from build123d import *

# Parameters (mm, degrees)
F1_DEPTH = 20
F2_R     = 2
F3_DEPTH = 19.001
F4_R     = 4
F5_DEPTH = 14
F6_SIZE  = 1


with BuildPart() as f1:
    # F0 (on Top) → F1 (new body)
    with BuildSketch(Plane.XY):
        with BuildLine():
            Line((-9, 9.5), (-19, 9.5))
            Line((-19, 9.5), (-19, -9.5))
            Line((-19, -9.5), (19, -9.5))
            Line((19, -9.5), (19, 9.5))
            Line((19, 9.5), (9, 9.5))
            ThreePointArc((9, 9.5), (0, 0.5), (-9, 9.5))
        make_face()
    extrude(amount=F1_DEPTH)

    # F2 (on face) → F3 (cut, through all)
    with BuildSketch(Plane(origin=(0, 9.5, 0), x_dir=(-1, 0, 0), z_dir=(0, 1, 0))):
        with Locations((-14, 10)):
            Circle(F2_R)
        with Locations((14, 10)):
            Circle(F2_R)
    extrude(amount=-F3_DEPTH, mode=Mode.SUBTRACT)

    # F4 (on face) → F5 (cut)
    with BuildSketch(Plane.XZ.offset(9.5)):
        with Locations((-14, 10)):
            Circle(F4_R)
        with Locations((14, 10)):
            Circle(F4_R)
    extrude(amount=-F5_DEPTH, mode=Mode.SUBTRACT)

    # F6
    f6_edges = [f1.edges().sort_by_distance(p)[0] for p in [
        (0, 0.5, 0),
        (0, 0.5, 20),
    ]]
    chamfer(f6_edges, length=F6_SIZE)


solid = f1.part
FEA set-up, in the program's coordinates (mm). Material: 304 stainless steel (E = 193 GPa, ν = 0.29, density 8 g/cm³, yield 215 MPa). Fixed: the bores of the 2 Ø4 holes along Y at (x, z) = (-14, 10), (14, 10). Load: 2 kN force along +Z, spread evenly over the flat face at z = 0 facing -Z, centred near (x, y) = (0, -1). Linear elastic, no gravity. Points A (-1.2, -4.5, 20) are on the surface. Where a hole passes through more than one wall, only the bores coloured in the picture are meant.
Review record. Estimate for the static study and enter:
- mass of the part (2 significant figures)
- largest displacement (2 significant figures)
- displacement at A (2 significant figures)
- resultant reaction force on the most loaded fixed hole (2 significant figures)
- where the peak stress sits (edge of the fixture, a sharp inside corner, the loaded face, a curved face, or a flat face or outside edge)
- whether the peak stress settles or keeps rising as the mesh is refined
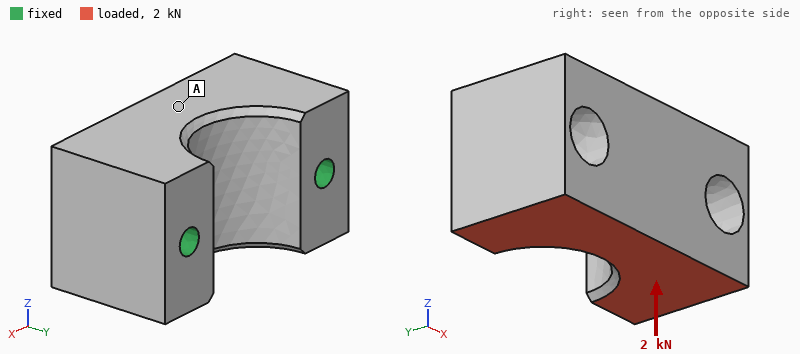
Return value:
83 g
11 µm
8.8 µm
1.0 kN
edge of the fixture
keeps rising
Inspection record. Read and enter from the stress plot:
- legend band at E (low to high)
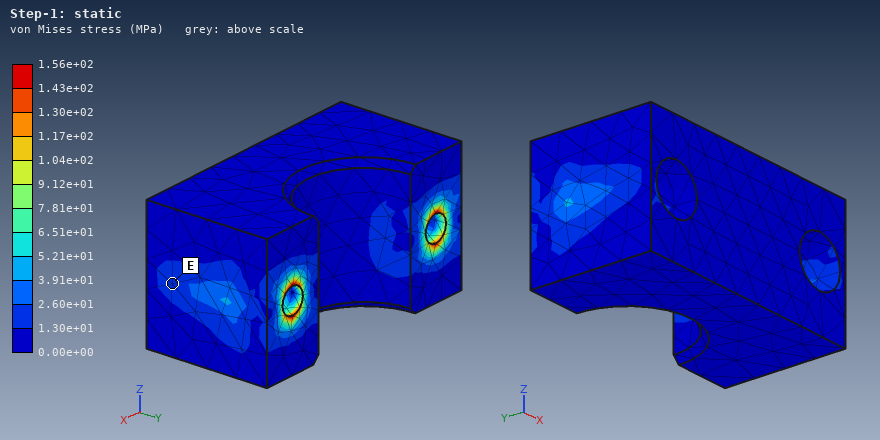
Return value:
1.30e+01 to 2.60e+01 MPa
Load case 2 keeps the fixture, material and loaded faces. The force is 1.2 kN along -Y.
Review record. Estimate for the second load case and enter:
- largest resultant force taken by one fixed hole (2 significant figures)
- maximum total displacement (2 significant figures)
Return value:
610 N
7.7 µm
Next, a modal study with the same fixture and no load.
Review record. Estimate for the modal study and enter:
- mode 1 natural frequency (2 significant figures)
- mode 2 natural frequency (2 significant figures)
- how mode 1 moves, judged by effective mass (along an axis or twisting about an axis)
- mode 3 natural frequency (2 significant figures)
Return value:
8500 Hz
19 kHz
along Z
20 kHz
